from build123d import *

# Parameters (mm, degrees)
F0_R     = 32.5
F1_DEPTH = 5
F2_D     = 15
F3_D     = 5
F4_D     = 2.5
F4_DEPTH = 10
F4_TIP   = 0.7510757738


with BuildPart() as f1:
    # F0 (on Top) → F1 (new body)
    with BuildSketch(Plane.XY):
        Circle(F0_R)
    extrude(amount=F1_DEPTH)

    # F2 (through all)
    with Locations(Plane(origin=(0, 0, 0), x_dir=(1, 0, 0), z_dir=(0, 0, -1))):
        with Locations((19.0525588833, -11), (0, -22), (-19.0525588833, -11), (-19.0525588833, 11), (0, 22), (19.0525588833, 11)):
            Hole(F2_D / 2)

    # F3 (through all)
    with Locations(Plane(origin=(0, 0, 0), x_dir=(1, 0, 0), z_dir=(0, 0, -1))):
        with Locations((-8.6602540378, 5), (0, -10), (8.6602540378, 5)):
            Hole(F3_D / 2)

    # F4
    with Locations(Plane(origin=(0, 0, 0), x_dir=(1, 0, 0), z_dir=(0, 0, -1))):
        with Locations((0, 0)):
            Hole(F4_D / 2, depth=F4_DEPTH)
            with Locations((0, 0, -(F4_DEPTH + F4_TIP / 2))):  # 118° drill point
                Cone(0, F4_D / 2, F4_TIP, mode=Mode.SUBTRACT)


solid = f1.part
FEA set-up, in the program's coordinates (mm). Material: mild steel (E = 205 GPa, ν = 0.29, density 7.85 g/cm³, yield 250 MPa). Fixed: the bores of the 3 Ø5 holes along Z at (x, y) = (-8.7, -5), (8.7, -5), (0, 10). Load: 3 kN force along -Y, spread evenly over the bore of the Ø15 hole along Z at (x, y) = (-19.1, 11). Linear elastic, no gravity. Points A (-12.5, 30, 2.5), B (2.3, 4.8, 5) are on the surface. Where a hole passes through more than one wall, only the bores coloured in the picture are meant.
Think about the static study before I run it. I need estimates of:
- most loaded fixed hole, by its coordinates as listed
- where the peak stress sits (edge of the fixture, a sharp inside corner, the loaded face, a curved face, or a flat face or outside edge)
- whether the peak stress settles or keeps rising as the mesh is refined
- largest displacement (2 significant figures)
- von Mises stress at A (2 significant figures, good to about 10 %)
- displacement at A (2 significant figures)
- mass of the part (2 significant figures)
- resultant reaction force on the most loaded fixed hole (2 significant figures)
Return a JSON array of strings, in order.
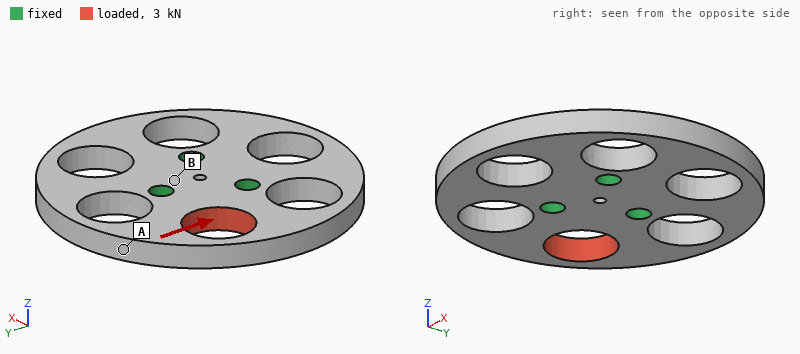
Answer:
["(-8.7, -5)", "edge of the fixture", "keeps rising", "16 µm", "35 MPa", "12 µm", "86 g", "2.8 kN"]
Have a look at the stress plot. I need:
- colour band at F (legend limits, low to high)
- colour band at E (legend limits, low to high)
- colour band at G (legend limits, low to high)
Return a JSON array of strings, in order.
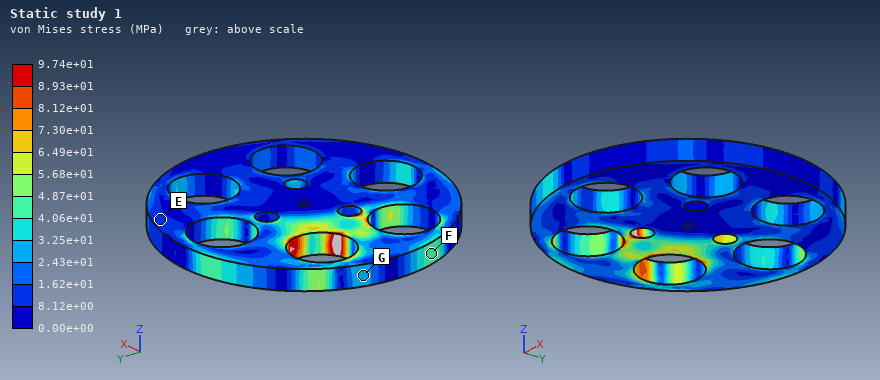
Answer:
["4.06e+01 to 4.87e+01 MPa", "8.12e+00 to 1.62e+01 MPa", "2.43e+01 to 3.25e+01 MPa"]
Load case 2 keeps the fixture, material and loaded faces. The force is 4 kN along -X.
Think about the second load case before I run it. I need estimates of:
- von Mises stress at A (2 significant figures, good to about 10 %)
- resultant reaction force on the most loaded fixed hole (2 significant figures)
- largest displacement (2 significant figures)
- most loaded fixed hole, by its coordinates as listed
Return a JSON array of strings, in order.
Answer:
["27 MPa", "3.2 kN", "15 µm", "(0, 10)"]
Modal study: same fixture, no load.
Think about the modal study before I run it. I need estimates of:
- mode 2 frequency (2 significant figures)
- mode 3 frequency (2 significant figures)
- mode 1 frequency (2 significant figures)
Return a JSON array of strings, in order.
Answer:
["5400 Hz", "5500 Hz", "5400 Hz"]
